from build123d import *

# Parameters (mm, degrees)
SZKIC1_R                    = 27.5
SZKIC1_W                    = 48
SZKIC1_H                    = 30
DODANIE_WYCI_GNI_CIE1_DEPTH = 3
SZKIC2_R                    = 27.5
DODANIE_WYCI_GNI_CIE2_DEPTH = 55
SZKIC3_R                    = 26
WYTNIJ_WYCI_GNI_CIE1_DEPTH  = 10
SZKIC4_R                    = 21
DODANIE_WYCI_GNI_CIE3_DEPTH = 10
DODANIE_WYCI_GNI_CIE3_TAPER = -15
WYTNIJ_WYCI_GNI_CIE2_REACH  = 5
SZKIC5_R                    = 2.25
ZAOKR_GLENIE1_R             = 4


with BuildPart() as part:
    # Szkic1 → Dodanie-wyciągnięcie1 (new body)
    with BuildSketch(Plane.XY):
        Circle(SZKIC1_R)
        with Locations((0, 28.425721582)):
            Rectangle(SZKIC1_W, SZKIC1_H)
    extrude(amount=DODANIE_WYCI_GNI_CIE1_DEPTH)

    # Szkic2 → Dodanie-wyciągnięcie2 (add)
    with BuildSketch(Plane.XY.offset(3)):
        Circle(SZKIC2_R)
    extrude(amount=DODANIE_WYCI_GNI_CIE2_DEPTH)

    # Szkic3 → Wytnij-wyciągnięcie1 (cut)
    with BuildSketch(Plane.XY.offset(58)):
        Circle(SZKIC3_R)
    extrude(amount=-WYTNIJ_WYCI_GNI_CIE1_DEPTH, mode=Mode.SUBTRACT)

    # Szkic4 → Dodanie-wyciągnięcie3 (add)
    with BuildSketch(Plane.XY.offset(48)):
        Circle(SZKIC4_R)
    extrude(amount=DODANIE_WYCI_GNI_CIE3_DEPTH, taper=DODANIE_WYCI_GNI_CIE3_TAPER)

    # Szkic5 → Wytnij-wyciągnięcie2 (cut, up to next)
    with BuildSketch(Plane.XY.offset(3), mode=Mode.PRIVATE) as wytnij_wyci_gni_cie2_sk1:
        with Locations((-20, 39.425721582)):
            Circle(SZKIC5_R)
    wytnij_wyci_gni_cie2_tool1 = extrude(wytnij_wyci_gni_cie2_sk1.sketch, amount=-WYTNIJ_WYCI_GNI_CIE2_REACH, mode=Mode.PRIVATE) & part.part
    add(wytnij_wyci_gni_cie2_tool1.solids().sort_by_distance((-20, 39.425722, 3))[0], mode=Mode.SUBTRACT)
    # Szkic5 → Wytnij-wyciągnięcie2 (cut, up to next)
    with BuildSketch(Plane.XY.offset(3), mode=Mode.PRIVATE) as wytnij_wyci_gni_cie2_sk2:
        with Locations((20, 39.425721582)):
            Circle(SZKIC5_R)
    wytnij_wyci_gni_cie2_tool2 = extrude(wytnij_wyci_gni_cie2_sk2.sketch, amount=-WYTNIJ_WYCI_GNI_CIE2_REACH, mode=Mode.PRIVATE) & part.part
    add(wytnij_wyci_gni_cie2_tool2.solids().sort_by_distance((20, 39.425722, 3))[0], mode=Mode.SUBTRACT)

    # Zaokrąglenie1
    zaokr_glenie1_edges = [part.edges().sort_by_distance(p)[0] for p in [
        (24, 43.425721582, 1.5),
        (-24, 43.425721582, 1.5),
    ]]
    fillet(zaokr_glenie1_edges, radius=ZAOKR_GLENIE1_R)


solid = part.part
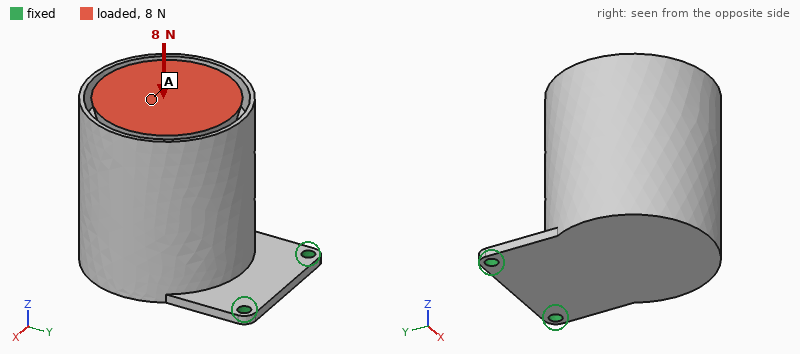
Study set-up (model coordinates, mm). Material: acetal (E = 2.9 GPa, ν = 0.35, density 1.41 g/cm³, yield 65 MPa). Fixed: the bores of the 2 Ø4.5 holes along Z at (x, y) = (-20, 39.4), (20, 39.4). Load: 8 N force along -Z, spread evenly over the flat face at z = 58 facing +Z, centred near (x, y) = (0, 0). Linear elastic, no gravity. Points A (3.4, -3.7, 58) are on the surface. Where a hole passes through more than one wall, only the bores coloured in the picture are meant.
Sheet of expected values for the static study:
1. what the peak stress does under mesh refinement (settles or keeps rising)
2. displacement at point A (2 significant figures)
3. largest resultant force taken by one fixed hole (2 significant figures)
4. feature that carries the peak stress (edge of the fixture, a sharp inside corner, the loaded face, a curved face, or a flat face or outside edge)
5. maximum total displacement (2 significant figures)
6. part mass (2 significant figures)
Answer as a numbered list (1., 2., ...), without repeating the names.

1. keeps rising
2. 0.89 mm
3. 4.2 N
4. edge of the fixture
5. 1.1 mm
6. 190 g
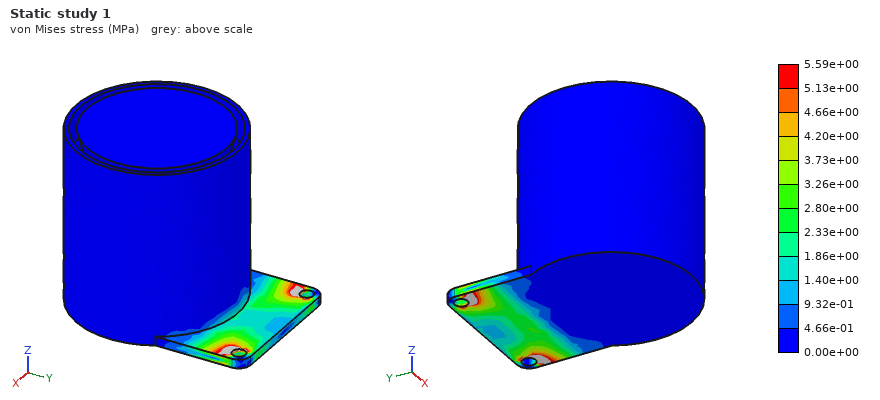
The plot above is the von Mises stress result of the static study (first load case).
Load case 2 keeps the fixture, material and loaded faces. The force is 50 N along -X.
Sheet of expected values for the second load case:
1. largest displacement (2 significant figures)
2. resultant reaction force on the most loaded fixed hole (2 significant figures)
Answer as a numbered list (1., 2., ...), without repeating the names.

1. 1.2 mm
2. 95 N
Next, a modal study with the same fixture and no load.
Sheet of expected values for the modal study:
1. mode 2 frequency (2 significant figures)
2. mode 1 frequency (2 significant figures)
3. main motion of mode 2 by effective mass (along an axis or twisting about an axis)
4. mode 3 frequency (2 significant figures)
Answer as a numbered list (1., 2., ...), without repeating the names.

1. 130 Hz
2. 35 Hz
3. along X
4. 370 Hz
